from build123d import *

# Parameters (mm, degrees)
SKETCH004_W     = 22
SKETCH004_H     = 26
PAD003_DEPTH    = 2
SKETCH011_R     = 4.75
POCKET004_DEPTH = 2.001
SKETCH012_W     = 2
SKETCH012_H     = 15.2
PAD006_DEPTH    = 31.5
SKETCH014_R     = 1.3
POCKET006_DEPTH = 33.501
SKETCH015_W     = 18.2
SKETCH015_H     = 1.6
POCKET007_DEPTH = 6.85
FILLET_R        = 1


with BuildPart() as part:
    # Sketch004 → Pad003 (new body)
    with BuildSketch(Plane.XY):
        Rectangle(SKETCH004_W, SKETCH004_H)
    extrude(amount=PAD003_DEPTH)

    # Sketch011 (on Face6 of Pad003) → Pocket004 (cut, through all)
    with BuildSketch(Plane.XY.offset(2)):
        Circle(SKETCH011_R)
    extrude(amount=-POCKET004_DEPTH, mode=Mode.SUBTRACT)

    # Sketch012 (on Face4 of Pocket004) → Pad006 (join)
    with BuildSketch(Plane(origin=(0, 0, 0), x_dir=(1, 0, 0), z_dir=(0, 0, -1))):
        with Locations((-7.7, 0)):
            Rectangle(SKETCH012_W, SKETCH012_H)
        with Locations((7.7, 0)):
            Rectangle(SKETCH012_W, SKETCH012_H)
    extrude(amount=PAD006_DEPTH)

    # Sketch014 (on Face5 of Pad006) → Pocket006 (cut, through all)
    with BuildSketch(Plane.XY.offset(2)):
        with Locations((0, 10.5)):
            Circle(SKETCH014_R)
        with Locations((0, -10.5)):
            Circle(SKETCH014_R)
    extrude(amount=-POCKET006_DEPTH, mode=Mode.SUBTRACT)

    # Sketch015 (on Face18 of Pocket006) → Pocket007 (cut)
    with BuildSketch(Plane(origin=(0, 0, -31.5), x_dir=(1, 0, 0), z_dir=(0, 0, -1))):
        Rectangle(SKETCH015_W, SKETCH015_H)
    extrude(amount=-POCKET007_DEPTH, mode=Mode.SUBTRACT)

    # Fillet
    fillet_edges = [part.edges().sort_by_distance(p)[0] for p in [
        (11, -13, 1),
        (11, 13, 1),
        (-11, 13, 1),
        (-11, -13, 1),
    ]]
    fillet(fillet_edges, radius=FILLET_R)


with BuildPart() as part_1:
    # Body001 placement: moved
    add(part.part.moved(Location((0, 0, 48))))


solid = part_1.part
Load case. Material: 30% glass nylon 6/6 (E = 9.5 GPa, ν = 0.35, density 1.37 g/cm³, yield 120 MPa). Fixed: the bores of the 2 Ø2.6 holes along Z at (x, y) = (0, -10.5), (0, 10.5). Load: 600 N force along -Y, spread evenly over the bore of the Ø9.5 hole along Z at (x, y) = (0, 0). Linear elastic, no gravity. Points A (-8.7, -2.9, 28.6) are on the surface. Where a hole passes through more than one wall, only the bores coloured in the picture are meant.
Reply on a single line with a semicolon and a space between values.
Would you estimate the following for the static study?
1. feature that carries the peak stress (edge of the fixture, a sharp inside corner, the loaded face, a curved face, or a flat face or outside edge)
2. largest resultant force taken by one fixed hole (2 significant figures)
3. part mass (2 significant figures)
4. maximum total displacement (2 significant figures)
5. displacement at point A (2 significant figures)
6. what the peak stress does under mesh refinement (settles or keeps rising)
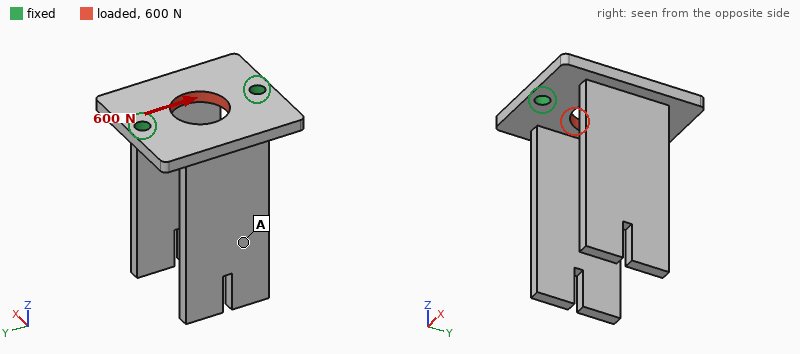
edge of the fixture; 300 N; 3.9 g; 20 µm; 12 µm; keeps rising
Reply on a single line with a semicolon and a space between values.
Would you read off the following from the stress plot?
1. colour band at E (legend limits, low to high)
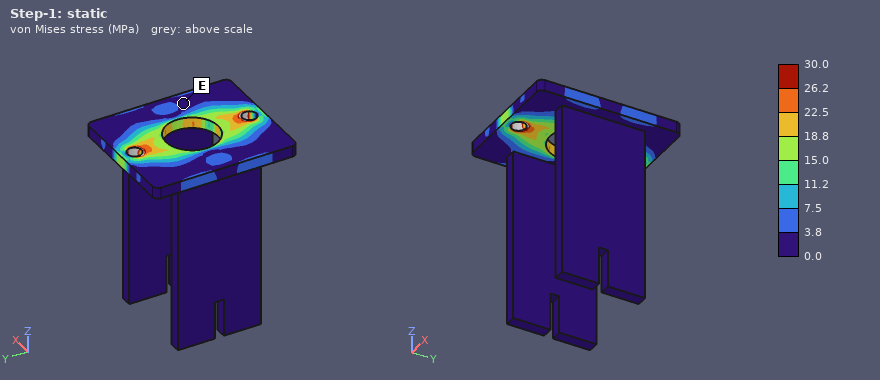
0.0 to 3.8 MPa
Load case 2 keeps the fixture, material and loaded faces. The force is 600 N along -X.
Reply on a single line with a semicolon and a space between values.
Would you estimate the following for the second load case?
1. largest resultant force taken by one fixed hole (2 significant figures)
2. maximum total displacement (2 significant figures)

300 N; 37 µm
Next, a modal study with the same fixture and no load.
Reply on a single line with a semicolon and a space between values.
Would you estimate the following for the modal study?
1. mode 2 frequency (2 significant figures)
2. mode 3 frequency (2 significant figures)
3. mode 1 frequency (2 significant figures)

640 Hz; 2100 Hz; 640 Hz
